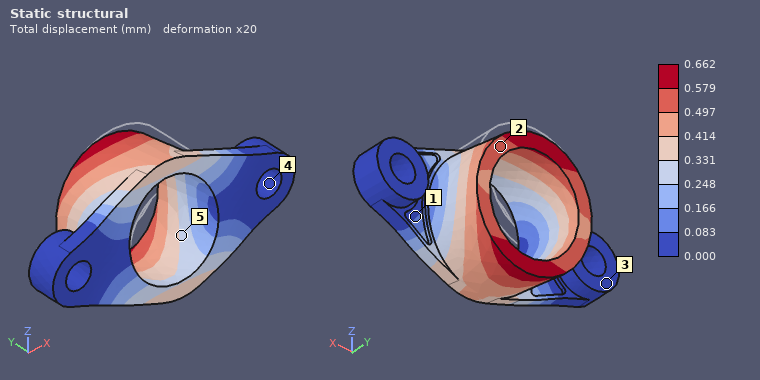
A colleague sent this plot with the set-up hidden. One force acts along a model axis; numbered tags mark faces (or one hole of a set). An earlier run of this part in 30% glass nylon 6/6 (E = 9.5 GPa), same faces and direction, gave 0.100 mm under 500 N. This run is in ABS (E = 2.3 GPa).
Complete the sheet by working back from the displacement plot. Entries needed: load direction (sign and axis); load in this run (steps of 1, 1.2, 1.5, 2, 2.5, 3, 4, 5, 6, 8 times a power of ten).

-Z
800 N
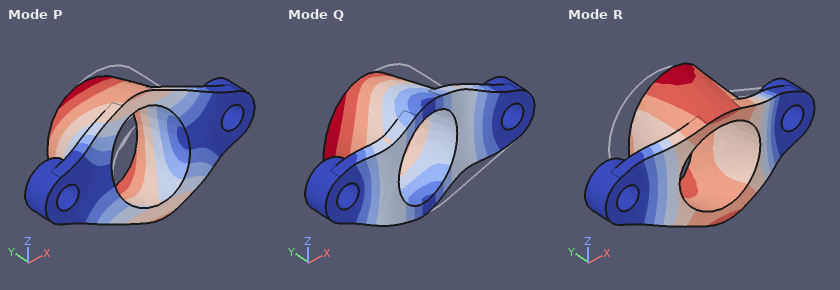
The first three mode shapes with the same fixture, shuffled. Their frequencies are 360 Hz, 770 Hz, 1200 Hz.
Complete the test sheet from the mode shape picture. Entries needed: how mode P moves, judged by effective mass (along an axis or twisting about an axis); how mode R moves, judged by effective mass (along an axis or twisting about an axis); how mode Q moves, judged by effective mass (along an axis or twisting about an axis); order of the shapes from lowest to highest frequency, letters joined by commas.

along Z
along Y
along X
P, R, Q
